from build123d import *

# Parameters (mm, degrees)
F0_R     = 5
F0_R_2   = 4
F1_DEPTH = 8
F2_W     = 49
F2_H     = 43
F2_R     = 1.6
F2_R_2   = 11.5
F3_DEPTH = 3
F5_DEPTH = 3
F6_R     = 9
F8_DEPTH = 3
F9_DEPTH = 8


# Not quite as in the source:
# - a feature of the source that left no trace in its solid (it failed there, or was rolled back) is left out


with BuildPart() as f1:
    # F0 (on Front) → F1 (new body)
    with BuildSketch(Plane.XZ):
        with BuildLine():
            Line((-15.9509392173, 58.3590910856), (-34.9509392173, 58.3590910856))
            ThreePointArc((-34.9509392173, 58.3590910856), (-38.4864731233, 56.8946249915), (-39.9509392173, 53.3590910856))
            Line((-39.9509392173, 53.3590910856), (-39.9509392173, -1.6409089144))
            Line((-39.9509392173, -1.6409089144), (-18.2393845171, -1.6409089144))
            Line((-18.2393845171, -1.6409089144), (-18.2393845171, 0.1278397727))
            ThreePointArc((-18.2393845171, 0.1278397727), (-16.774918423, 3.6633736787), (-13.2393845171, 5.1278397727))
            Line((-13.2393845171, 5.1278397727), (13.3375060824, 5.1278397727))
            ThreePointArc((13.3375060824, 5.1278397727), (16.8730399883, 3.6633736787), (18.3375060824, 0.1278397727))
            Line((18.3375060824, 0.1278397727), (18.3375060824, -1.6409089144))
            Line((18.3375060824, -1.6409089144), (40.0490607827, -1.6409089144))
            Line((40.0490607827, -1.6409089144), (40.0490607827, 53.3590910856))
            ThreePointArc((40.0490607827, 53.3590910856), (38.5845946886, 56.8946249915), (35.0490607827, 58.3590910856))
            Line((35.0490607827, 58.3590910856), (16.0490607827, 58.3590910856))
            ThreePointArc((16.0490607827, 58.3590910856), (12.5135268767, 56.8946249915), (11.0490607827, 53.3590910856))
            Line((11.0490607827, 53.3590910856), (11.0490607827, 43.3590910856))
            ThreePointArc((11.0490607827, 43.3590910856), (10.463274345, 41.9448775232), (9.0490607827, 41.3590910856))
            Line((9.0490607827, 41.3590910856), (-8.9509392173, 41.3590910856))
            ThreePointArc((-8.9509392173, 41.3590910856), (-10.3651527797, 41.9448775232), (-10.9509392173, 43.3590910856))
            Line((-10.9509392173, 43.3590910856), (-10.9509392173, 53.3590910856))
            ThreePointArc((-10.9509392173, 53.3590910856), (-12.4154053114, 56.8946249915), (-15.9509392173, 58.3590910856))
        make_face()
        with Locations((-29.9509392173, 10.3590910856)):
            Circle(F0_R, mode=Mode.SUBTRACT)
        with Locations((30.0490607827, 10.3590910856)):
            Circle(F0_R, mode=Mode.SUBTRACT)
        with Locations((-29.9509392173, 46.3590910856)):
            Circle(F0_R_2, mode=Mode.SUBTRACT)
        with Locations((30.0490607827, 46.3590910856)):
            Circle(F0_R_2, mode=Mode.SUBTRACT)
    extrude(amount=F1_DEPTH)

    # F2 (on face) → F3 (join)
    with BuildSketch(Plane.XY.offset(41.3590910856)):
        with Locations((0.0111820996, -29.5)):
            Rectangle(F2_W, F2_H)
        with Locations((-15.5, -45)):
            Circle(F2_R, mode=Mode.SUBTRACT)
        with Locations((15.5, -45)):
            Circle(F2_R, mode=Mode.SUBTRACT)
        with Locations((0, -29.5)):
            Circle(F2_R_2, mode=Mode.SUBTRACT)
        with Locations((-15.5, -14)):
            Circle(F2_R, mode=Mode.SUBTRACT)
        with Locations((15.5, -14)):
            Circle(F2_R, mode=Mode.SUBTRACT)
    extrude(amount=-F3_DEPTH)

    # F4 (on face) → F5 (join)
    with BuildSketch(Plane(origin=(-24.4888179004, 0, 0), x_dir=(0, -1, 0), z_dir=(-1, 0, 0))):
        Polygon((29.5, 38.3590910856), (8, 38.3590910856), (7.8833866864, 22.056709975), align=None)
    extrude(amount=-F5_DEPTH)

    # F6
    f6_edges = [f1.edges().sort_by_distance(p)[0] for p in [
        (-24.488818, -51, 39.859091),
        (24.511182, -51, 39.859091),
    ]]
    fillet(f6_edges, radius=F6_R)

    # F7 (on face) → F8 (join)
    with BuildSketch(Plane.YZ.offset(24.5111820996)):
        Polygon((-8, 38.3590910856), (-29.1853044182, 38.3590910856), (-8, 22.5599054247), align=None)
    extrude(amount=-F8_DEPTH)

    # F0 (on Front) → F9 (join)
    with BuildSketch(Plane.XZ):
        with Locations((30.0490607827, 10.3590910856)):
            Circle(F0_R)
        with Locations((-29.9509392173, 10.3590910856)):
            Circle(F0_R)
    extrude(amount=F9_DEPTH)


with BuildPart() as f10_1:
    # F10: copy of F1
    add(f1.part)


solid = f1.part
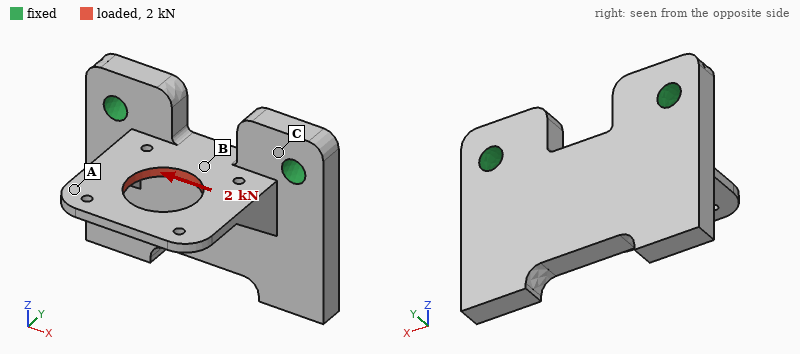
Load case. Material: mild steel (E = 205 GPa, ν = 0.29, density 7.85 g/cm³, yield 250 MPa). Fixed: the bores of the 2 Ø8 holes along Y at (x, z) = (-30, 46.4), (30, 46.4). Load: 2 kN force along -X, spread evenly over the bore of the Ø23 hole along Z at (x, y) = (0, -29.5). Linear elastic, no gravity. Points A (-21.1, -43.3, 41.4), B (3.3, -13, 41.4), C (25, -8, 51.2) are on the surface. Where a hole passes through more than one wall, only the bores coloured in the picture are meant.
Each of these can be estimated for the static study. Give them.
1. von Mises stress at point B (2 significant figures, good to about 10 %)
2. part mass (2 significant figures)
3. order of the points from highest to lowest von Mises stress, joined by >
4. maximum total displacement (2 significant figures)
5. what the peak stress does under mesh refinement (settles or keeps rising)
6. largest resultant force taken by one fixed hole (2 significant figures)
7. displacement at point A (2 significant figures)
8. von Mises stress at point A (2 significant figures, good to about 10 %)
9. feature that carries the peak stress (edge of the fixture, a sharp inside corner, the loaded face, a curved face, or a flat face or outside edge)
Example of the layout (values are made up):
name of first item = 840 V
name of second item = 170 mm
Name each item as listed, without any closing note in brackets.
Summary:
von Mises stress at point B = 34 MPa
part mass = 300 g
order of the points from highest to lowest von Mises stress, joined by > = B > A > C
maximum total displacement = 20 µm
what the peak stress does under mesh refinement = keeps rising
largest resultant force taken by one fixed hole = 1.4 kN
displacement at point A = 18 µm
von Mises stress at point A = 14 MPa
feature that carries the peak stress = a sharp inside corner
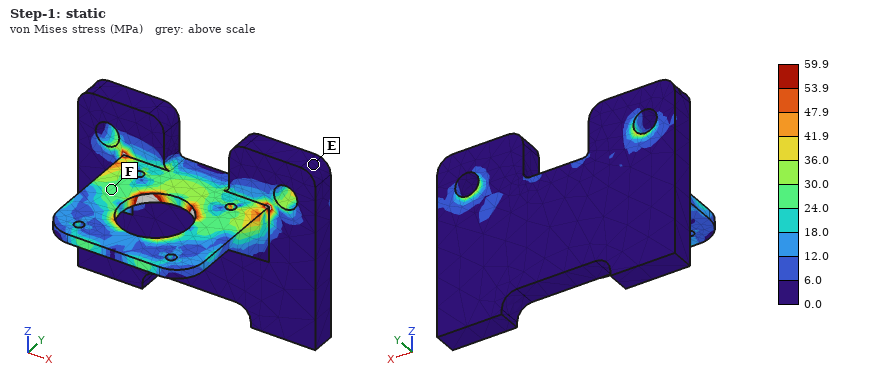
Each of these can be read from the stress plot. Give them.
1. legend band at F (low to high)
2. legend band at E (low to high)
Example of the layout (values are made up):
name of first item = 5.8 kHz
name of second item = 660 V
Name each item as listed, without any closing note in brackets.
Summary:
legend band at F = 24.0 to 30.0 MPa
legend band at E = 0.0 to 6.0 MPa
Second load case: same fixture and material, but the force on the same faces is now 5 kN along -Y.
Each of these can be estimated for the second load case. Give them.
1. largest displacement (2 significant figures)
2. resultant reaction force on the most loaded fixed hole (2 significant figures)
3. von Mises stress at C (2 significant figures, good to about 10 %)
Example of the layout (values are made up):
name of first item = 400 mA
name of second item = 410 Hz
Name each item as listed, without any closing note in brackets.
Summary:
largest displacement = 21 µm
resultant reaction force on the most loaded fixed hole = 2.6 kN
von Mises stress at C = 26 MPa
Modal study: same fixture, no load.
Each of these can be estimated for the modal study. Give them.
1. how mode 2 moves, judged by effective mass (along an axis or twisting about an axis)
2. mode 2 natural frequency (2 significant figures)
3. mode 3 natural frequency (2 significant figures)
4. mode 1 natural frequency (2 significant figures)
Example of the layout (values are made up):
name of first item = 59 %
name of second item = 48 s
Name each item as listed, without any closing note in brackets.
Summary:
how mode 2 moves, judged by effective mass = along Y
mode 2 natural frequency = 3100 Hz
mode 3 natural frequency = 4400 Hz
mode 1 natural frequency = 2100 Hz
